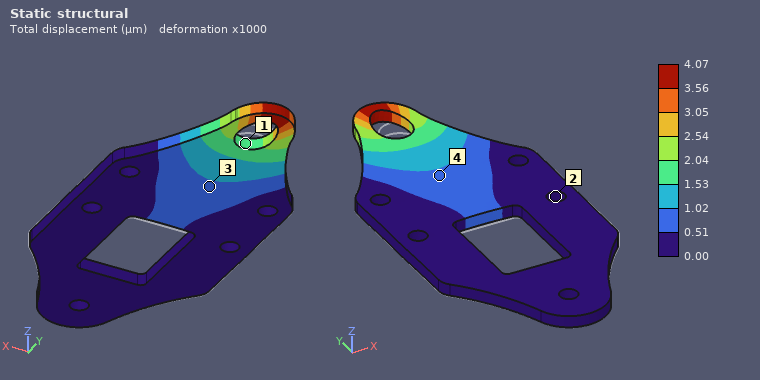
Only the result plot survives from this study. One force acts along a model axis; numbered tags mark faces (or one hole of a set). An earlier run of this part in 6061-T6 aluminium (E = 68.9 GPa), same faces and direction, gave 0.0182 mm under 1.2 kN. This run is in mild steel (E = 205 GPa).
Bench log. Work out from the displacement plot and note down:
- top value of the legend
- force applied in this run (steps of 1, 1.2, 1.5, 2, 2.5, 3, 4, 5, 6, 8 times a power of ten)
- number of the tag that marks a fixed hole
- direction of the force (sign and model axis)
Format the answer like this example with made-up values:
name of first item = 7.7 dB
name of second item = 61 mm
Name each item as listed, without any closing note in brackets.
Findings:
top value of the legend = 4.07 µm
force applied in this run = 800 N
number of the tag that marks a fixed hole = 2
direction of the force = +Y
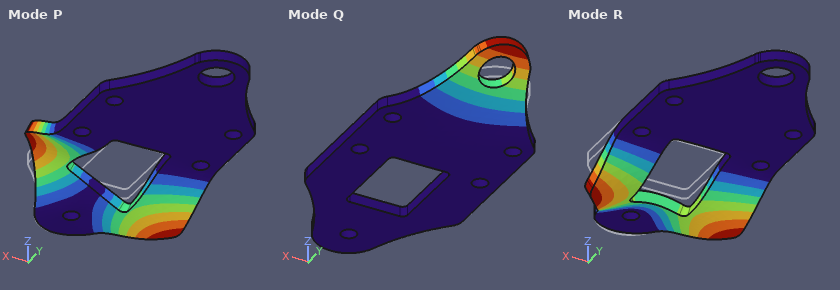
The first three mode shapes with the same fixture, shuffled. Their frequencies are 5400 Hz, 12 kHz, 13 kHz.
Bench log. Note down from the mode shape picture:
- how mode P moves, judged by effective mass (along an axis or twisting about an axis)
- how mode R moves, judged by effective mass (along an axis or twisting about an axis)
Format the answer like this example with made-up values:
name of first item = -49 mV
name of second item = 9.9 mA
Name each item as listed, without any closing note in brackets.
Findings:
how mode P moves, judged by effective mass = twisting about Y
how mode R moves, judged by effective mass = along Z
